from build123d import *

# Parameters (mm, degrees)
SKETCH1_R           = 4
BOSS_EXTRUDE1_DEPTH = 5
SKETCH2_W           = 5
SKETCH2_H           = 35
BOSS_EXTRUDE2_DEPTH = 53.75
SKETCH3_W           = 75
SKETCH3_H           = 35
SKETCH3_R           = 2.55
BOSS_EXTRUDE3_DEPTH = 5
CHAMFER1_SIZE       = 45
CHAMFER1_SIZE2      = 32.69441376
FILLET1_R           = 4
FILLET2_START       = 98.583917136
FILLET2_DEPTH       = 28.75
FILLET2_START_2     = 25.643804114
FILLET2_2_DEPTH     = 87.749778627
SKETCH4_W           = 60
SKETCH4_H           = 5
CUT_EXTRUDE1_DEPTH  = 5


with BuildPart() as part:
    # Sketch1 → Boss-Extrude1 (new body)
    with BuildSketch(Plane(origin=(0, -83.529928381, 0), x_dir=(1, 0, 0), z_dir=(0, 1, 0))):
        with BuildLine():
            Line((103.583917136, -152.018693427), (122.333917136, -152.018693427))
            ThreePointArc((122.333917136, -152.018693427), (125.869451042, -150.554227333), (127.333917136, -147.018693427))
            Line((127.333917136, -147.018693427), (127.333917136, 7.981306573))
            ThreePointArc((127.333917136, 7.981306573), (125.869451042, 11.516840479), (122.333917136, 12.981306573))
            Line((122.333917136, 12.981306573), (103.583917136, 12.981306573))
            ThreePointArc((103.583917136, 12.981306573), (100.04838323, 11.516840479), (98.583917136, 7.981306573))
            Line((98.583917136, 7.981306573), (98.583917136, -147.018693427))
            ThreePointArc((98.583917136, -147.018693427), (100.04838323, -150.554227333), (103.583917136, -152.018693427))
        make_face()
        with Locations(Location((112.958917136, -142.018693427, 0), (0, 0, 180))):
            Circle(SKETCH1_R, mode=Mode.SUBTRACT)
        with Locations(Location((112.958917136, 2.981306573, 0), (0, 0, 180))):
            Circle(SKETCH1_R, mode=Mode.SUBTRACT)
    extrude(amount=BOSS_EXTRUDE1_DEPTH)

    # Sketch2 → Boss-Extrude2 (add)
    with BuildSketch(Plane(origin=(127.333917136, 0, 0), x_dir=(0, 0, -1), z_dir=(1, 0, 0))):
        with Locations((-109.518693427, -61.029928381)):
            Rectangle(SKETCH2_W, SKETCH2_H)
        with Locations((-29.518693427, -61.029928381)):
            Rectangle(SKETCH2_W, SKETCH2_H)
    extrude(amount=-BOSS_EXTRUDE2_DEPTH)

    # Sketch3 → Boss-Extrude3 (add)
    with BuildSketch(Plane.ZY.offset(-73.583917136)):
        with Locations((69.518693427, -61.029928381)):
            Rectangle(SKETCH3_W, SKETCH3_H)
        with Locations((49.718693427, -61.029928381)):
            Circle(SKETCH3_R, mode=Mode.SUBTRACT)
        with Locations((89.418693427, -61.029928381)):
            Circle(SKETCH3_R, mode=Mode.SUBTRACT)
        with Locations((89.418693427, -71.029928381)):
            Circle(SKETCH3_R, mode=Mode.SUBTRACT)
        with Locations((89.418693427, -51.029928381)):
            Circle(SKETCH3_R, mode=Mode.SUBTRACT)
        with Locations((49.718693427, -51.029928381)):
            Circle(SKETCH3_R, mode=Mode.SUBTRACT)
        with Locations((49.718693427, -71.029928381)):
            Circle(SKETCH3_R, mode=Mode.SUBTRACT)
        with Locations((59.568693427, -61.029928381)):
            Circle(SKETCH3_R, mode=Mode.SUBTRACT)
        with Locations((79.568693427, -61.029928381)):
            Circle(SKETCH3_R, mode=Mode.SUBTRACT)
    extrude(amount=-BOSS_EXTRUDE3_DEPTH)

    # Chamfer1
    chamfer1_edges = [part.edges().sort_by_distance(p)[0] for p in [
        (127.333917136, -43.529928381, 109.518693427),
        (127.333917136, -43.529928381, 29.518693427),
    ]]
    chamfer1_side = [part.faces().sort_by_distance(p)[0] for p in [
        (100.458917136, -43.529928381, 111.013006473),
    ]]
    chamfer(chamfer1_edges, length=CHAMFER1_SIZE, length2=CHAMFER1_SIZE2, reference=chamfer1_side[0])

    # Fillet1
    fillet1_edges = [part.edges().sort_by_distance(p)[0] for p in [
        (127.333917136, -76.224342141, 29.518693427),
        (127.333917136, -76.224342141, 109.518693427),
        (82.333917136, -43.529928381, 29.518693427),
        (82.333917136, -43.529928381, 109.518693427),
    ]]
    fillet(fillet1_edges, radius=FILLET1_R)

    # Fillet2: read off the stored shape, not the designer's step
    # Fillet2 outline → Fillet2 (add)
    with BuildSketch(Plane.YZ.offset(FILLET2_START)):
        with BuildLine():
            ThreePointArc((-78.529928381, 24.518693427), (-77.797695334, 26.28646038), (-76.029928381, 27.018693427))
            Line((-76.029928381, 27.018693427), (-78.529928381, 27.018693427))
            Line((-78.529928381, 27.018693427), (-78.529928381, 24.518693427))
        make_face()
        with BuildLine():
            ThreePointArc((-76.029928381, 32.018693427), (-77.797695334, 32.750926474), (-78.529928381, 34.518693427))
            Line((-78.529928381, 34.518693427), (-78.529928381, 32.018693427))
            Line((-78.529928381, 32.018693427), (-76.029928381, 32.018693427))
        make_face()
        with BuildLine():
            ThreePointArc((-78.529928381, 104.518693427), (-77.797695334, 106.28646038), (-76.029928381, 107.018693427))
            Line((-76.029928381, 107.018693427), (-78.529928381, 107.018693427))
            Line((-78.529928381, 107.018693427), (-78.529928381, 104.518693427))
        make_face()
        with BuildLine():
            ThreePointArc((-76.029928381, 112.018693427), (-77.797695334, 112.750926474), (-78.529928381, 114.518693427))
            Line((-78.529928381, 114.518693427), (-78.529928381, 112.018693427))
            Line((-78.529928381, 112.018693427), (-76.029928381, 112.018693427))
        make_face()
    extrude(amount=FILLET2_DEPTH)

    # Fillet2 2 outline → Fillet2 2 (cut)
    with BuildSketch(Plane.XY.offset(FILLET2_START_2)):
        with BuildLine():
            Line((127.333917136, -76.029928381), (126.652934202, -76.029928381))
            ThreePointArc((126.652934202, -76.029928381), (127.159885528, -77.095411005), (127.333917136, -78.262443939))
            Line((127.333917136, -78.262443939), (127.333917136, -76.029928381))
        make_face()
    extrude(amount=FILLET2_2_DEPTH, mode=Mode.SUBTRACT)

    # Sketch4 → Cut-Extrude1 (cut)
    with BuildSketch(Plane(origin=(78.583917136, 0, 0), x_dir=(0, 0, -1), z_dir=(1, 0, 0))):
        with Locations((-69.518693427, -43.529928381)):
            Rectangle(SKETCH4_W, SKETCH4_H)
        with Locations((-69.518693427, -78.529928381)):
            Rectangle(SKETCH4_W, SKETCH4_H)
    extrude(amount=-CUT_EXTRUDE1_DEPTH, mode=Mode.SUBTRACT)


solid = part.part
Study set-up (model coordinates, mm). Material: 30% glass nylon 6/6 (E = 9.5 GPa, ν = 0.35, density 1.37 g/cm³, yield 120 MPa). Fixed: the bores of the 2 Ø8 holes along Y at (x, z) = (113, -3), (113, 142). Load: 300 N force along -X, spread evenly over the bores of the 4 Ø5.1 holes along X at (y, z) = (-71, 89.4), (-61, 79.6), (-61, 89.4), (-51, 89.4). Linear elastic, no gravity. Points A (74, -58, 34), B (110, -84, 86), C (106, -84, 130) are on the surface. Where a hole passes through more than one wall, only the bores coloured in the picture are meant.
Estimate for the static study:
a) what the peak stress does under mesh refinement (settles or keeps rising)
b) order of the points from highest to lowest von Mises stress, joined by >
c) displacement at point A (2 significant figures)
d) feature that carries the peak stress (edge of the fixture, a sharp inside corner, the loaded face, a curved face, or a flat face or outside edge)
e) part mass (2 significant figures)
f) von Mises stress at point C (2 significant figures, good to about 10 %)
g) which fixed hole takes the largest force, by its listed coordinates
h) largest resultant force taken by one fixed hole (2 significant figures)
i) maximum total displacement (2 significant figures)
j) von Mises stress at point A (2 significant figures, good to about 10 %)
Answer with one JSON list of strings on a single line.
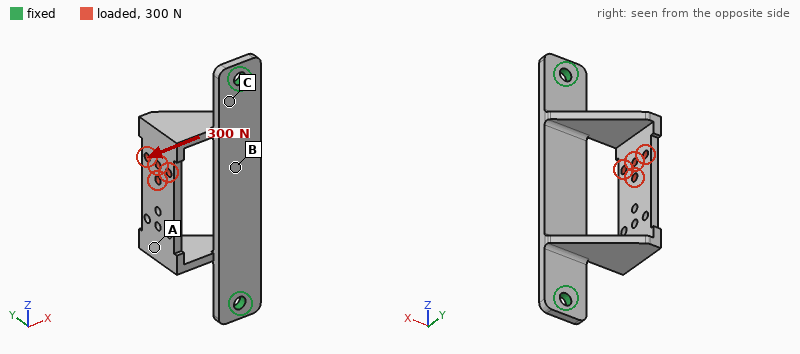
["keeps rising", "C > A > B", "0.84 mm", "edge of the fixture", "62 g", "19 MPa", "(113, 142)", "200 N", "1.4 mm", "9.5 MPa"]
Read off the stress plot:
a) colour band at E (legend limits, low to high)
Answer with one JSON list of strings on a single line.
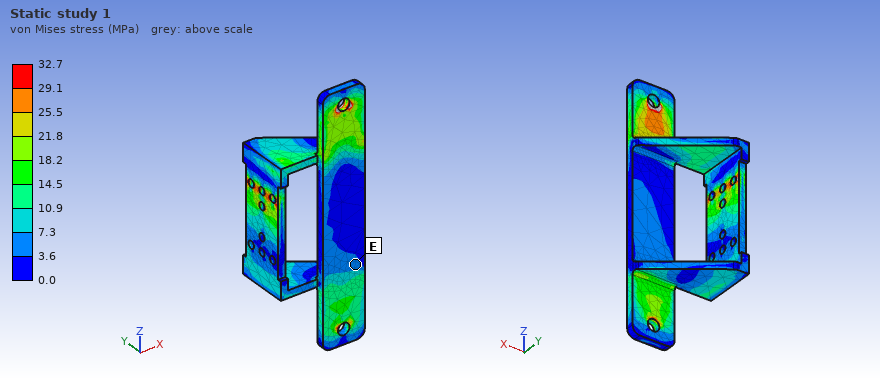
["3.6 to 7.3 MPa"]
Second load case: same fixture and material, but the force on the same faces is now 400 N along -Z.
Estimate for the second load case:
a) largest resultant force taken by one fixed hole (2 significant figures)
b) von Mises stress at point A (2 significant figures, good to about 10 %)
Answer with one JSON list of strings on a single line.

["240 N", "13 MPa"]
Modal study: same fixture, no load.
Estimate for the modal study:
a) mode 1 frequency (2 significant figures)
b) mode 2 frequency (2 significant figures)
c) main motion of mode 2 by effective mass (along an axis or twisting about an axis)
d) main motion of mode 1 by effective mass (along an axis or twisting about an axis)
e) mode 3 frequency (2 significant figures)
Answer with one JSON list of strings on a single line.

["400 Hz", "780 Hz", "along Y", "along Y", "880 Hz"]
